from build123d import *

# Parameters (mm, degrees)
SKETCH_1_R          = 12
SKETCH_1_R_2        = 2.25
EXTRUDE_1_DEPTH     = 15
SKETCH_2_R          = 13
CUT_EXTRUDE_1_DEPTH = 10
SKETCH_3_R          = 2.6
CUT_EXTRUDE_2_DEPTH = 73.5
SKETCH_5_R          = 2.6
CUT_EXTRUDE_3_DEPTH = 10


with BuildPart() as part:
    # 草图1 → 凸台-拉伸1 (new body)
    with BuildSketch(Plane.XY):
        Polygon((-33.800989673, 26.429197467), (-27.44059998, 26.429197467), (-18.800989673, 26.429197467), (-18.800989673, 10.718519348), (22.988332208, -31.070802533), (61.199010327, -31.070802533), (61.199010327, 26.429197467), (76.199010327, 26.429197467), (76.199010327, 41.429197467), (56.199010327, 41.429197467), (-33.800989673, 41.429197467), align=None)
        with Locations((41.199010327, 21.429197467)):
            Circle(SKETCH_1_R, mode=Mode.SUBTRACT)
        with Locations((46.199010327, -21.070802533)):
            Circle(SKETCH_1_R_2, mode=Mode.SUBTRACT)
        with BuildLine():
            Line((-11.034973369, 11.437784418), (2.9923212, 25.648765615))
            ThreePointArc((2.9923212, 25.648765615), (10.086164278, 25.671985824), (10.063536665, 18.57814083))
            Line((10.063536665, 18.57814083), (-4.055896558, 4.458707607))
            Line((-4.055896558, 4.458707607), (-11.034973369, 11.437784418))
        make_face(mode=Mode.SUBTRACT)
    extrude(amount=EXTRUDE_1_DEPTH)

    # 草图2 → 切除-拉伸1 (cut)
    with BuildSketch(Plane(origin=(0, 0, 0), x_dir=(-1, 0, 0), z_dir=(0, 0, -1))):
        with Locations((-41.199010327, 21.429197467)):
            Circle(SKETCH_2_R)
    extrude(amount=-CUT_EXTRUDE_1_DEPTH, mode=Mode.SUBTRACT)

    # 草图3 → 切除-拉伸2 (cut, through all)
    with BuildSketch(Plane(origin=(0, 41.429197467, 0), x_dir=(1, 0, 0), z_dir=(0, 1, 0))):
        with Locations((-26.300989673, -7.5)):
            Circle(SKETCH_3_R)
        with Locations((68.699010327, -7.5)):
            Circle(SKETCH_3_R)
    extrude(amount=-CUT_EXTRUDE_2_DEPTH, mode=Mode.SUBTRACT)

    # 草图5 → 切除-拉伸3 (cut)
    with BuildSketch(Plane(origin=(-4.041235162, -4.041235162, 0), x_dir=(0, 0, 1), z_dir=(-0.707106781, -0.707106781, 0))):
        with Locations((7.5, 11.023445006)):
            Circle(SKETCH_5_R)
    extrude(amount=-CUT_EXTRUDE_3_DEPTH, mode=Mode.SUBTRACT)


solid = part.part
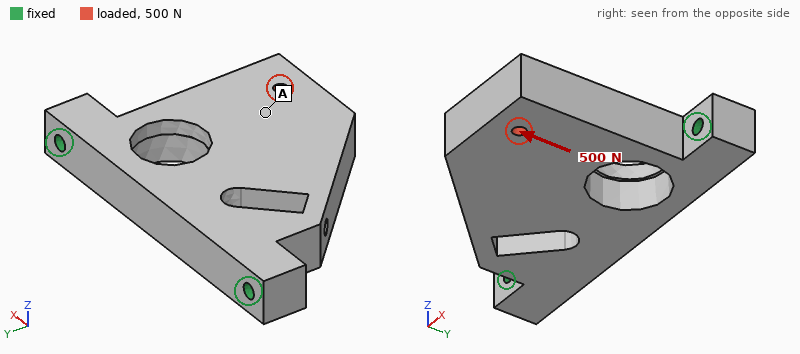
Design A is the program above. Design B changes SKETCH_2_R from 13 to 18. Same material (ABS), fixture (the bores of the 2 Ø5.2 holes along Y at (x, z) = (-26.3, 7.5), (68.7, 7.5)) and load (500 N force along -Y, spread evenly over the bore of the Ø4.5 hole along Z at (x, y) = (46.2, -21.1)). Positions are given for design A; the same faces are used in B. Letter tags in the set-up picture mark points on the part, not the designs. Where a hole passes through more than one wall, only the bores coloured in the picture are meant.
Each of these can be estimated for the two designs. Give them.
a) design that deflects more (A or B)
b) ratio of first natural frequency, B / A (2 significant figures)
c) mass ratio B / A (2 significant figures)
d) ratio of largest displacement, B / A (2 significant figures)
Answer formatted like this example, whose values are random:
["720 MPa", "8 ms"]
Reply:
["B", "0.91", "0.93", "2.0"]
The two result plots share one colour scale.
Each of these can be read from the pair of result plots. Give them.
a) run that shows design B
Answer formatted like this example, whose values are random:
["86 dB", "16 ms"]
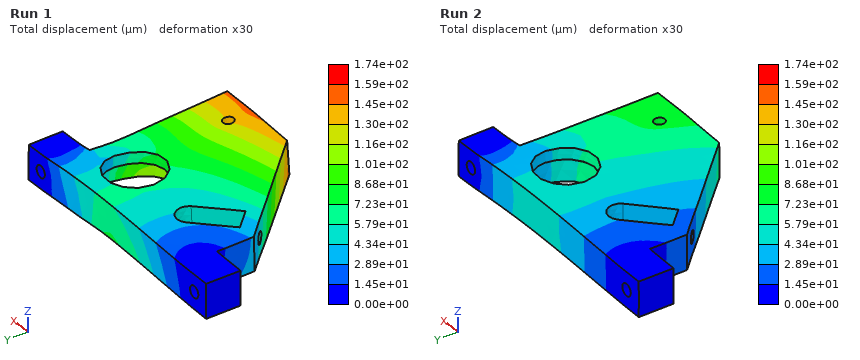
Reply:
["Run 1"]
